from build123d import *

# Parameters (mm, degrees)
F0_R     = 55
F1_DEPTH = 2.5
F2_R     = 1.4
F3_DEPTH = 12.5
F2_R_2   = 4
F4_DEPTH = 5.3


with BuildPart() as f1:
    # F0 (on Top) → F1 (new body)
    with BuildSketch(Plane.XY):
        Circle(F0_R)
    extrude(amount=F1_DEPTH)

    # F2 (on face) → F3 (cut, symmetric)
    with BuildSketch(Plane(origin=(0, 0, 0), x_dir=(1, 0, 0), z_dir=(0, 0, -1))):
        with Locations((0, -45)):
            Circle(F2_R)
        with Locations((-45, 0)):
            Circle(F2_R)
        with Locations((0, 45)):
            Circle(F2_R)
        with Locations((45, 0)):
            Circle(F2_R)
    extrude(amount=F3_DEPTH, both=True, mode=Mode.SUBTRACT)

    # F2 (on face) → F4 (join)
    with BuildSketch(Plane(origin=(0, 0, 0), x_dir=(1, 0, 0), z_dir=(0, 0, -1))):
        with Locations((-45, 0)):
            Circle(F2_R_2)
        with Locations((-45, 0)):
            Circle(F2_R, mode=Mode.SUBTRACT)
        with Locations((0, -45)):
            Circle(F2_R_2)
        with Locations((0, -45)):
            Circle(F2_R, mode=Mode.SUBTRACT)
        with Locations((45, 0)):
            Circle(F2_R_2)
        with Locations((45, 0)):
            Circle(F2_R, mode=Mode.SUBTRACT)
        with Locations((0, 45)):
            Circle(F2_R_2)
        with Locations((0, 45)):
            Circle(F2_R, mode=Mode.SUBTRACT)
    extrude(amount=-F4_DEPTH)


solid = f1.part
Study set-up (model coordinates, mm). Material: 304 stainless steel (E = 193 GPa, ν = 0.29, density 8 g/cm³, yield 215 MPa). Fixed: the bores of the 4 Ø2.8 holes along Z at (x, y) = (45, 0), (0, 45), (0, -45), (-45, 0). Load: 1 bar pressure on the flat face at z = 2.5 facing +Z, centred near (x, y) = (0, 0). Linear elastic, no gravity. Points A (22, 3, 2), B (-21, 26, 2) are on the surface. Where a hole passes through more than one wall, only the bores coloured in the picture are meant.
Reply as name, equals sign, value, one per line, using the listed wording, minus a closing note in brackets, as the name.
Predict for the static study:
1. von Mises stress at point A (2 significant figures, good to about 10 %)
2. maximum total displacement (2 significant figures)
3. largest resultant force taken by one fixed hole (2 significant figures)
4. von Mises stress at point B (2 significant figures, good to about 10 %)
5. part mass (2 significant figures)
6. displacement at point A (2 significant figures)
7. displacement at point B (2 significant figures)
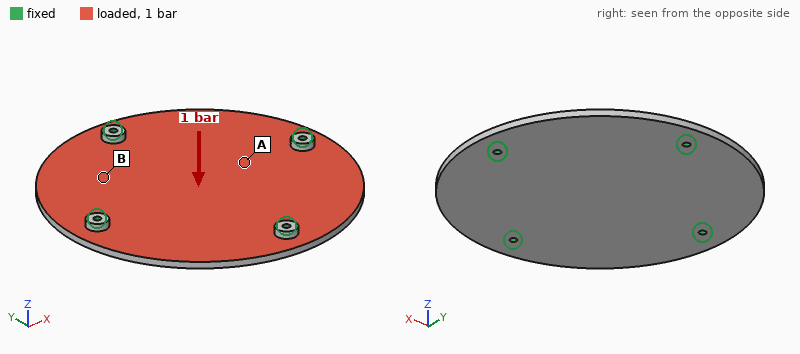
von Mises stress at point A = 10 MPa
maximum total displacement = 33 µm
largest resultant force taken by one fixed hole = 240 N
von Mises stress at point B = 20 MPa
part mass = 190 g
displacement at point A = 22 µm
displacement at point B = 21 µm
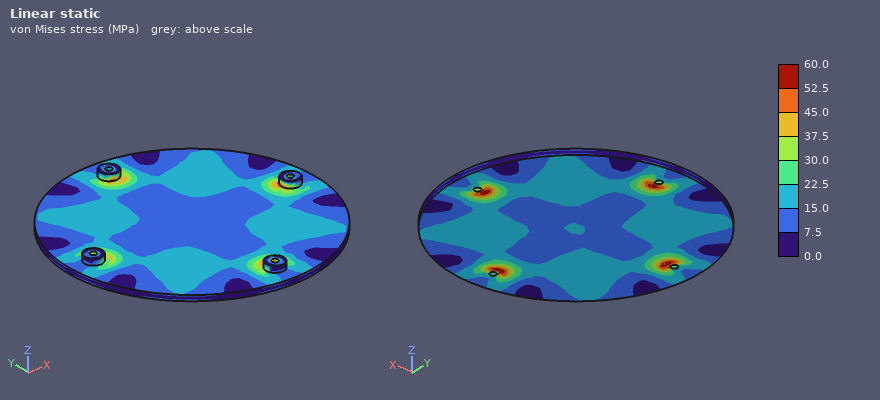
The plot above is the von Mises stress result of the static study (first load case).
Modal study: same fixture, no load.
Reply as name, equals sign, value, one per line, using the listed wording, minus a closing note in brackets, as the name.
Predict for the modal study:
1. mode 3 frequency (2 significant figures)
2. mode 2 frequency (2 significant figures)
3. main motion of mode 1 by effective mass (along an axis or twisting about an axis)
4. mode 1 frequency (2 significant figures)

mode 3 frequency = 2600 Hz
mode 2 frequency = 2500 Hz
main motion of mode 1 by effective mass = along Z
mode 1 frequency = 2300 Hz
